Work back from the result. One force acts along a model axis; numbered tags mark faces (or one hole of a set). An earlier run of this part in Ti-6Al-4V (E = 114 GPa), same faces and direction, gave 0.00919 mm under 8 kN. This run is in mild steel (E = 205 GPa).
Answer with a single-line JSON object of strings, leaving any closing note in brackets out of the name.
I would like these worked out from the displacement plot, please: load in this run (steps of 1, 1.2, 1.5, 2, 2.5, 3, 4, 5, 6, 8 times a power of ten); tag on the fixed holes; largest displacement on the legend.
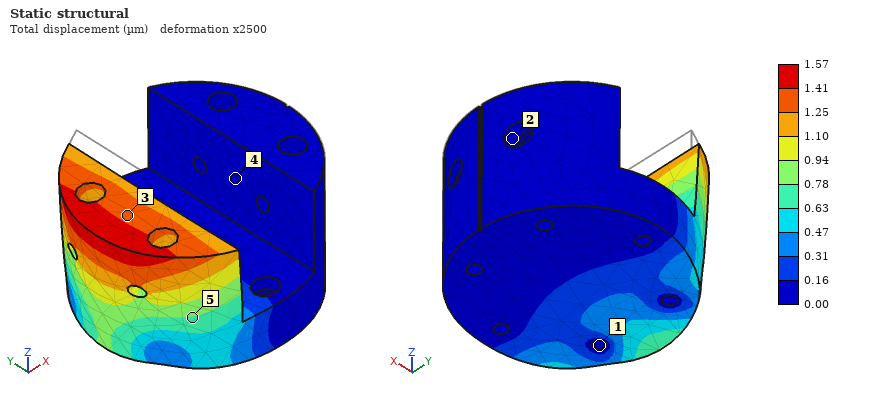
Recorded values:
{"load in this run": "2.5 kN", "tag on the fixed holes": "1", "largest displacement on the legend": "1.57 µm"}
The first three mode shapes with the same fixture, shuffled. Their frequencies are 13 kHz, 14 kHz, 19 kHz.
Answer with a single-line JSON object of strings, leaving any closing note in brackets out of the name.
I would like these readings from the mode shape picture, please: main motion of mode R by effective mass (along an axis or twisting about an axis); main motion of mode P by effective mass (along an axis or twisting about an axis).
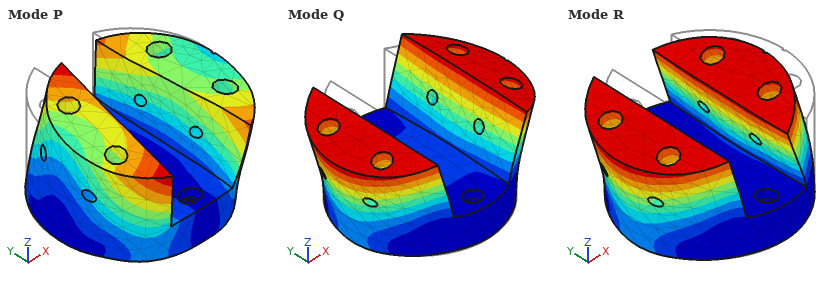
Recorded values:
{"main motion of mode R by effective mass": "along X", "main motion of mode P by effective mass": "along Y"}
